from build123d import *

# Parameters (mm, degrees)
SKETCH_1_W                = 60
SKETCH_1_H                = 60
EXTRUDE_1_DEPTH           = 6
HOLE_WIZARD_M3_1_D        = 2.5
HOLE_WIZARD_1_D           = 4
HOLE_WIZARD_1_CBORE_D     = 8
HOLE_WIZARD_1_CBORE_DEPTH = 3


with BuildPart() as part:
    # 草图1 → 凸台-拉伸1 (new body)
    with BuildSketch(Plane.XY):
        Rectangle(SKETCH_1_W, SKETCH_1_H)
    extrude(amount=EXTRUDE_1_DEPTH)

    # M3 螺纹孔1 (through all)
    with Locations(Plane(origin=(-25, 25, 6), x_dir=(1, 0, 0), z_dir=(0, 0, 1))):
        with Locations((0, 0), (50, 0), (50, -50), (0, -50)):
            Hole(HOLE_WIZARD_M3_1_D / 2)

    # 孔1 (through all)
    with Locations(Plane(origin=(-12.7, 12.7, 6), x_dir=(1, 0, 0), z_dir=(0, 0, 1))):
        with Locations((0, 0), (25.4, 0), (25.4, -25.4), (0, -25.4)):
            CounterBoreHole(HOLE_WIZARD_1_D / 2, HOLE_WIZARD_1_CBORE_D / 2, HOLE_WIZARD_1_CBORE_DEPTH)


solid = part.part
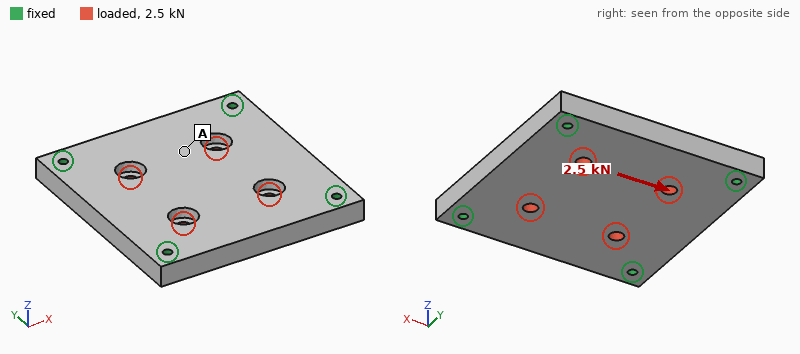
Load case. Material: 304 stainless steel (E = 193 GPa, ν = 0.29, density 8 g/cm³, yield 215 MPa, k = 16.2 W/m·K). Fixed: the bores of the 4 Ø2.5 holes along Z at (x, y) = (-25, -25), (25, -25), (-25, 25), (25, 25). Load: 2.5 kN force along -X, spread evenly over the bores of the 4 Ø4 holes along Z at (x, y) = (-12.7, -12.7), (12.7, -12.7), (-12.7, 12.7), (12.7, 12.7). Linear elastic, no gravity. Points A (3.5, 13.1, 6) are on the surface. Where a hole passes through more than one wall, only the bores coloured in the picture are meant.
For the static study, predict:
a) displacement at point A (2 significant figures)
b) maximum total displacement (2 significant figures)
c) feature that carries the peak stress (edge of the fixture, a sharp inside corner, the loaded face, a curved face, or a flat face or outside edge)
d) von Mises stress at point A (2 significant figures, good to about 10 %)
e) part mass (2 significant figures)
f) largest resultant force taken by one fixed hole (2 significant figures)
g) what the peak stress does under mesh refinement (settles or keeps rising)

1.00 µm
1.5 µm
edge of the fixture
4.3 MPa
170 g
670 N
keeps rising
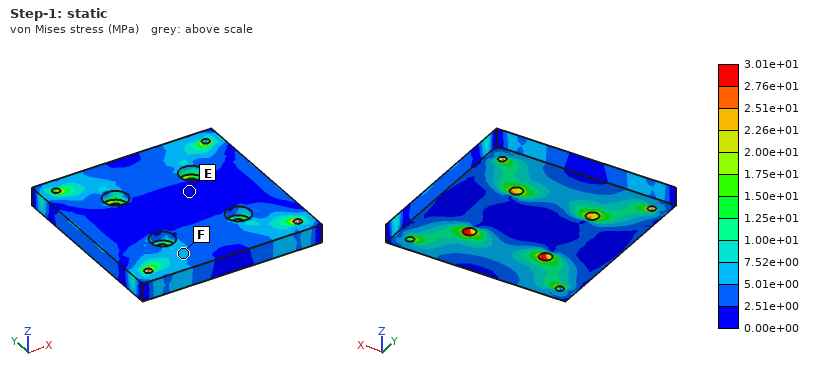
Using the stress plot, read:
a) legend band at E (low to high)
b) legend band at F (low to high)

0.00e+00 to 2.51e+00 MPa
5.01e+00 to 7.52e+00 MPa
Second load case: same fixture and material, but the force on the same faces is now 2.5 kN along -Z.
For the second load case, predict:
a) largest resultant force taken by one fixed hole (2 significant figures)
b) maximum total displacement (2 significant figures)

630 N
17 µm
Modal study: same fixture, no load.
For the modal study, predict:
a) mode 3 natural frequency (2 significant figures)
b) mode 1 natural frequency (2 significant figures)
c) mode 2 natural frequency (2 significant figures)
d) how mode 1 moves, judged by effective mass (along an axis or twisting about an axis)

11 kHz
6800 Hz
11 kHz
along Z
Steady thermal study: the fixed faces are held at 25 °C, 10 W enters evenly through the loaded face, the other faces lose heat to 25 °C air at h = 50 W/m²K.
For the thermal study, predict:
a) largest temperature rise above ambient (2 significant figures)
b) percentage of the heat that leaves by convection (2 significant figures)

23 K
44 %
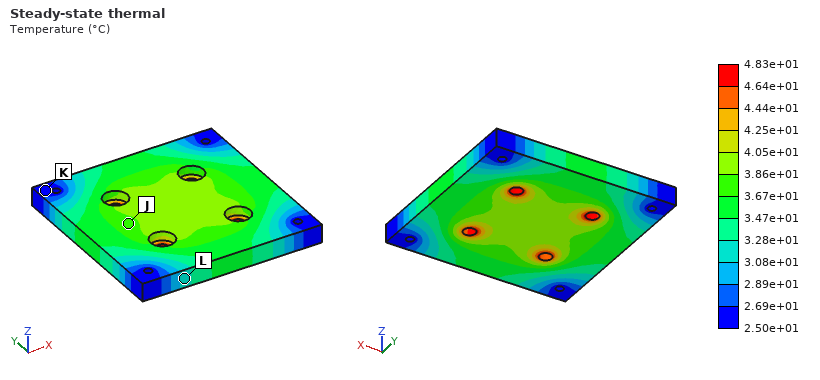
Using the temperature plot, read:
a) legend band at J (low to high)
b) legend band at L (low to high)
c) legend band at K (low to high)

3.67e+01 to 3.86e+01 °C
3.08e+01 to 3.28e+01 °C
2.50e+01 to 2.69e+01 °C
